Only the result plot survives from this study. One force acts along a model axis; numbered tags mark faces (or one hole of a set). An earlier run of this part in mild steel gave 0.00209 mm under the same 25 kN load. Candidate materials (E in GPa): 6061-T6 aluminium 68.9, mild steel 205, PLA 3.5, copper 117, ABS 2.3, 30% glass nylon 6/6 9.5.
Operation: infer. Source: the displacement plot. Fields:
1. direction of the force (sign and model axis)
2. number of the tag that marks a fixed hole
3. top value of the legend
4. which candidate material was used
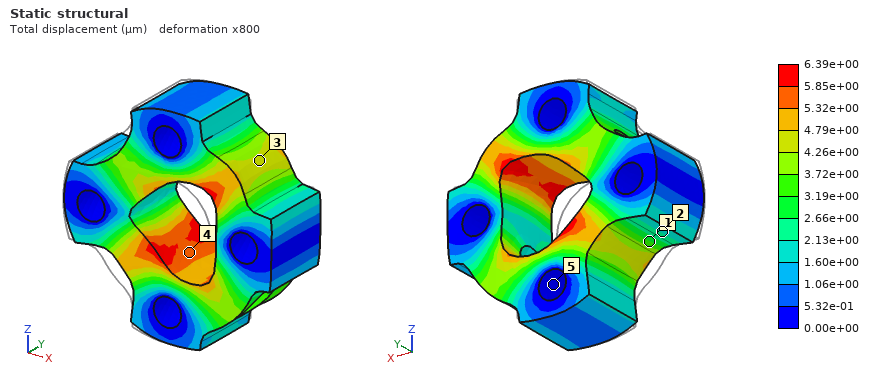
+X
5
6.39e+00 µm
6061-T6 aluminium
